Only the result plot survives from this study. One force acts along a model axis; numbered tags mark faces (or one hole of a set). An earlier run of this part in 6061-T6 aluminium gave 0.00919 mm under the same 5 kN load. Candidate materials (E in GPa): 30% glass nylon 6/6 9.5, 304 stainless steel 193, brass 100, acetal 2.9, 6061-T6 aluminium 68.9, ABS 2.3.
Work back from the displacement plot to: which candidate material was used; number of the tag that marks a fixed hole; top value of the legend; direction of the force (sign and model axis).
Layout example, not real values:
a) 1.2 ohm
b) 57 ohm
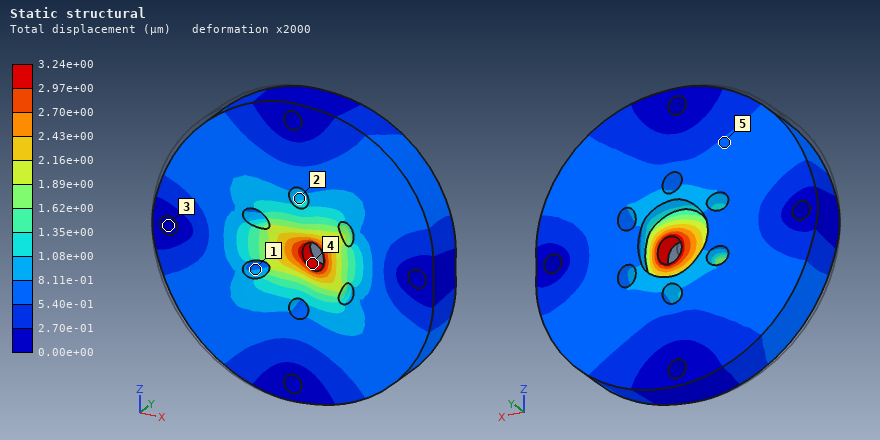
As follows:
a) 304 stainless steel
b) 3
c) 3.24e+00 µm
d) +X
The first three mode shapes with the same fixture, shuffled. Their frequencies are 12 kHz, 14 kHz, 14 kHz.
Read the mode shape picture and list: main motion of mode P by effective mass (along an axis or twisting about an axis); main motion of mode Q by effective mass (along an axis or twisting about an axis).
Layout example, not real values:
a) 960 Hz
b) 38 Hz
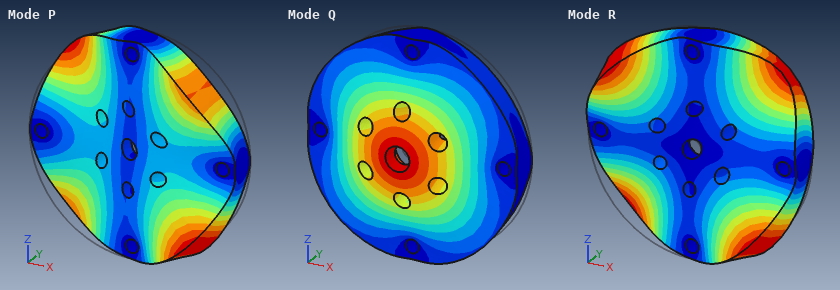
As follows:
a) twisting about Z
b) along Y
